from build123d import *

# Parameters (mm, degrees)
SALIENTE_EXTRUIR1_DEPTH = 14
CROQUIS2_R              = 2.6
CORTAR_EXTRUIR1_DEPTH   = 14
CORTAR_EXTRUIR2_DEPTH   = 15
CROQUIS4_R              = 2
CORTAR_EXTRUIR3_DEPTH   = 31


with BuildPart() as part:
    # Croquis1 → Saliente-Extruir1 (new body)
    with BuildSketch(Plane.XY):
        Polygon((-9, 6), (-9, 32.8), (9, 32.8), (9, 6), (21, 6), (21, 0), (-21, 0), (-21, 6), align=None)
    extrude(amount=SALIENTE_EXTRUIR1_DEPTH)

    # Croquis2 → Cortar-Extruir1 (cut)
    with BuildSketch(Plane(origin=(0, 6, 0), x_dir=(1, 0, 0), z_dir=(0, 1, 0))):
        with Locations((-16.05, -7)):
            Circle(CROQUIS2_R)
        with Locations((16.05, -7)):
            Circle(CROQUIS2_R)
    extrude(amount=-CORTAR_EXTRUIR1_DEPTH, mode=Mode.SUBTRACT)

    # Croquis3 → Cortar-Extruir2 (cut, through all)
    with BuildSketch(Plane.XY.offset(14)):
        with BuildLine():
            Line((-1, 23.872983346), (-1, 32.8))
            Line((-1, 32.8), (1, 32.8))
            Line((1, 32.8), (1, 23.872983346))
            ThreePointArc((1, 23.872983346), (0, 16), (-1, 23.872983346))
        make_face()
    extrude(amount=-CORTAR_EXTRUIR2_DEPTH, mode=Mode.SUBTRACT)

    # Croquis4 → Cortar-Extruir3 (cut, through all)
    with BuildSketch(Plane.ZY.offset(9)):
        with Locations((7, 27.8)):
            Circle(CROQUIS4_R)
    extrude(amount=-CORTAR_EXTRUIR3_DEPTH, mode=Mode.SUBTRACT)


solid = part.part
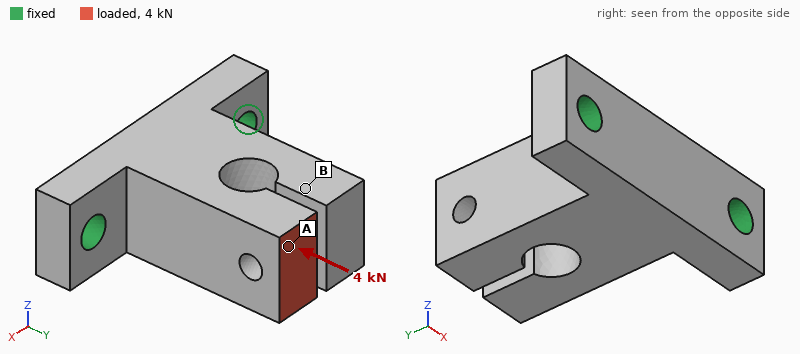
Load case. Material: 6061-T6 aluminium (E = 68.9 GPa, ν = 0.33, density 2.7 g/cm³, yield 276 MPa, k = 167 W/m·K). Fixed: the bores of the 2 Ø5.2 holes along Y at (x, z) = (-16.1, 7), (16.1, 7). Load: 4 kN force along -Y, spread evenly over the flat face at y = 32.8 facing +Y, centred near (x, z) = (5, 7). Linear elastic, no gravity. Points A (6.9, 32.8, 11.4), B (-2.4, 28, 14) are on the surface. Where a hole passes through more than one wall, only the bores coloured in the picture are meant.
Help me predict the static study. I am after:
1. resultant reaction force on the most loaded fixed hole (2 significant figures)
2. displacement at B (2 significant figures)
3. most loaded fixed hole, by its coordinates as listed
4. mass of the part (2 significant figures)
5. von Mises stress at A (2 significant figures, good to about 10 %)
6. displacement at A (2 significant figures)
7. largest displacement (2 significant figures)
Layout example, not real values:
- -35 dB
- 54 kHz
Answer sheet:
- 2.9 kN
- 22 µm
- (16.1, 7)
- 24 g
- 39 MPa
- 41 µm
- 59 µm
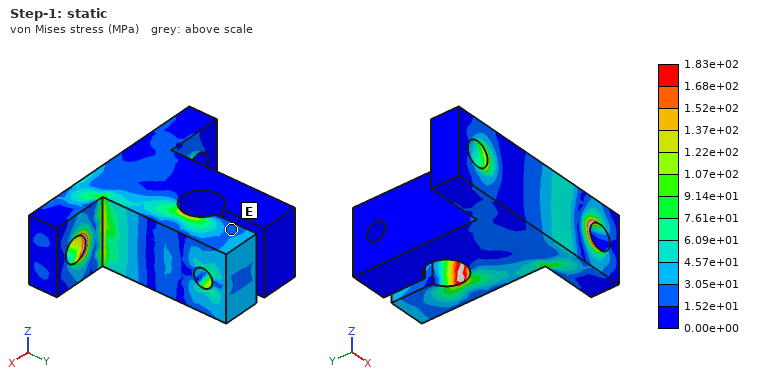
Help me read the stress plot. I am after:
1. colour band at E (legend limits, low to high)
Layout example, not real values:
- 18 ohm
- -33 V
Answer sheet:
- 1.52e+01 to 3.05e+01 MPa
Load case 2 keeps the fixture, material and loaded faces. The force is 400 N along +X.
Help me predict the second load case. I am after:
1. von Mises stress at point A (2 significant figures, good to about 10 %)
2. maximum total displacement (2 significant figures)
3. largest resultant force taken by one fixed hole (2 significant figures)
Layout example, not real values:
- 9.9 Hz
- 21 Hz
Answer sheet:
- 8.9 MPa
- 84 µm
- 570 N
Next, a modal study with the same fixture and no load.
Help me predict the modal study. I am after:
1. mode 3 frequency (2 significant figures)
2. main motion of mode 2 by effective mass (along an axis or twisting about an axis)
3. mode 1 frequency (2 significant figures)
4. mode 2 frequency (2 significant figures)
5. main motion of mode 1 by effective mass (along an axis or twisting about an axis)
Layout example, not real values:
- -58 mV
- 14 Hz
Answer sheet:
- 10 kHz
- along X
- 5100 Hz
- 8300 Hz
- along Z
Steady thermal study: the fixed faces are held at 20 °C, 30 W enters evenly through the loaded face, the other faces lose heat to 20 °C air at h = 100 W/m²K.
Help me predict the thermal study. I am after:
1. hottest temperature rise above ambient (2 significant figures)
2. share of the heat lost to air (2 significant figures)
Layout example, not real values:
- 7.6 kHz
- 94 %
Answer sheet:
- 54 K
- 18 %
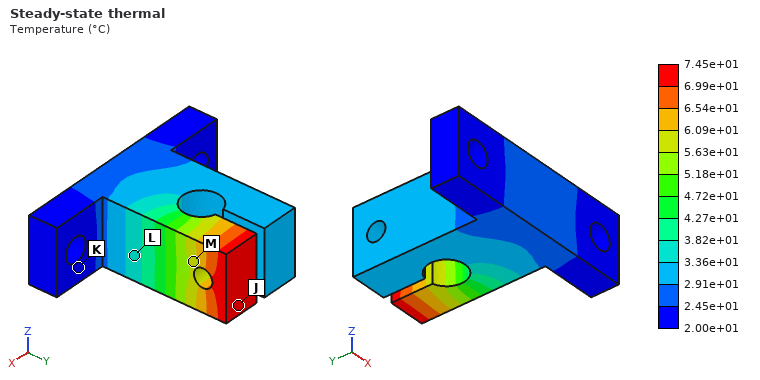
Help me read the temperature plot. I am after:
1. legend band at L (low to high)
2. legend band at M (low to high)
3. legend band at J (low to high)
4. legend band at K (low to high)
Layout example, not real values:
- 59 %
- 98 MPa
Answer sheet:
- 3.36e+01 to 3.82e+01 °C
- 5.63e+01 to 6.09e+01 °C
- 6.99e+01 to 7.45e+01 °C
- 2.00e+01 to 2.45e+01 °C
